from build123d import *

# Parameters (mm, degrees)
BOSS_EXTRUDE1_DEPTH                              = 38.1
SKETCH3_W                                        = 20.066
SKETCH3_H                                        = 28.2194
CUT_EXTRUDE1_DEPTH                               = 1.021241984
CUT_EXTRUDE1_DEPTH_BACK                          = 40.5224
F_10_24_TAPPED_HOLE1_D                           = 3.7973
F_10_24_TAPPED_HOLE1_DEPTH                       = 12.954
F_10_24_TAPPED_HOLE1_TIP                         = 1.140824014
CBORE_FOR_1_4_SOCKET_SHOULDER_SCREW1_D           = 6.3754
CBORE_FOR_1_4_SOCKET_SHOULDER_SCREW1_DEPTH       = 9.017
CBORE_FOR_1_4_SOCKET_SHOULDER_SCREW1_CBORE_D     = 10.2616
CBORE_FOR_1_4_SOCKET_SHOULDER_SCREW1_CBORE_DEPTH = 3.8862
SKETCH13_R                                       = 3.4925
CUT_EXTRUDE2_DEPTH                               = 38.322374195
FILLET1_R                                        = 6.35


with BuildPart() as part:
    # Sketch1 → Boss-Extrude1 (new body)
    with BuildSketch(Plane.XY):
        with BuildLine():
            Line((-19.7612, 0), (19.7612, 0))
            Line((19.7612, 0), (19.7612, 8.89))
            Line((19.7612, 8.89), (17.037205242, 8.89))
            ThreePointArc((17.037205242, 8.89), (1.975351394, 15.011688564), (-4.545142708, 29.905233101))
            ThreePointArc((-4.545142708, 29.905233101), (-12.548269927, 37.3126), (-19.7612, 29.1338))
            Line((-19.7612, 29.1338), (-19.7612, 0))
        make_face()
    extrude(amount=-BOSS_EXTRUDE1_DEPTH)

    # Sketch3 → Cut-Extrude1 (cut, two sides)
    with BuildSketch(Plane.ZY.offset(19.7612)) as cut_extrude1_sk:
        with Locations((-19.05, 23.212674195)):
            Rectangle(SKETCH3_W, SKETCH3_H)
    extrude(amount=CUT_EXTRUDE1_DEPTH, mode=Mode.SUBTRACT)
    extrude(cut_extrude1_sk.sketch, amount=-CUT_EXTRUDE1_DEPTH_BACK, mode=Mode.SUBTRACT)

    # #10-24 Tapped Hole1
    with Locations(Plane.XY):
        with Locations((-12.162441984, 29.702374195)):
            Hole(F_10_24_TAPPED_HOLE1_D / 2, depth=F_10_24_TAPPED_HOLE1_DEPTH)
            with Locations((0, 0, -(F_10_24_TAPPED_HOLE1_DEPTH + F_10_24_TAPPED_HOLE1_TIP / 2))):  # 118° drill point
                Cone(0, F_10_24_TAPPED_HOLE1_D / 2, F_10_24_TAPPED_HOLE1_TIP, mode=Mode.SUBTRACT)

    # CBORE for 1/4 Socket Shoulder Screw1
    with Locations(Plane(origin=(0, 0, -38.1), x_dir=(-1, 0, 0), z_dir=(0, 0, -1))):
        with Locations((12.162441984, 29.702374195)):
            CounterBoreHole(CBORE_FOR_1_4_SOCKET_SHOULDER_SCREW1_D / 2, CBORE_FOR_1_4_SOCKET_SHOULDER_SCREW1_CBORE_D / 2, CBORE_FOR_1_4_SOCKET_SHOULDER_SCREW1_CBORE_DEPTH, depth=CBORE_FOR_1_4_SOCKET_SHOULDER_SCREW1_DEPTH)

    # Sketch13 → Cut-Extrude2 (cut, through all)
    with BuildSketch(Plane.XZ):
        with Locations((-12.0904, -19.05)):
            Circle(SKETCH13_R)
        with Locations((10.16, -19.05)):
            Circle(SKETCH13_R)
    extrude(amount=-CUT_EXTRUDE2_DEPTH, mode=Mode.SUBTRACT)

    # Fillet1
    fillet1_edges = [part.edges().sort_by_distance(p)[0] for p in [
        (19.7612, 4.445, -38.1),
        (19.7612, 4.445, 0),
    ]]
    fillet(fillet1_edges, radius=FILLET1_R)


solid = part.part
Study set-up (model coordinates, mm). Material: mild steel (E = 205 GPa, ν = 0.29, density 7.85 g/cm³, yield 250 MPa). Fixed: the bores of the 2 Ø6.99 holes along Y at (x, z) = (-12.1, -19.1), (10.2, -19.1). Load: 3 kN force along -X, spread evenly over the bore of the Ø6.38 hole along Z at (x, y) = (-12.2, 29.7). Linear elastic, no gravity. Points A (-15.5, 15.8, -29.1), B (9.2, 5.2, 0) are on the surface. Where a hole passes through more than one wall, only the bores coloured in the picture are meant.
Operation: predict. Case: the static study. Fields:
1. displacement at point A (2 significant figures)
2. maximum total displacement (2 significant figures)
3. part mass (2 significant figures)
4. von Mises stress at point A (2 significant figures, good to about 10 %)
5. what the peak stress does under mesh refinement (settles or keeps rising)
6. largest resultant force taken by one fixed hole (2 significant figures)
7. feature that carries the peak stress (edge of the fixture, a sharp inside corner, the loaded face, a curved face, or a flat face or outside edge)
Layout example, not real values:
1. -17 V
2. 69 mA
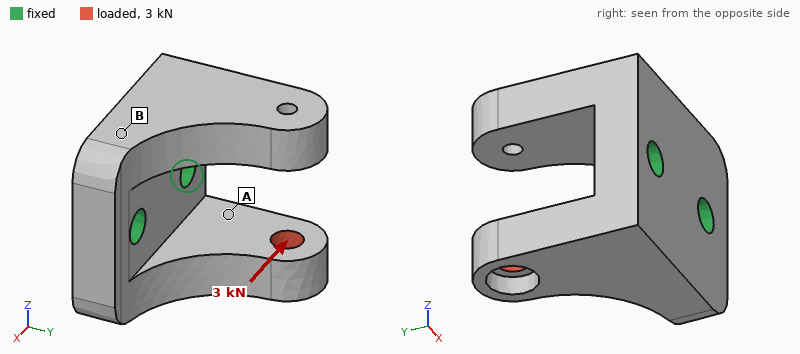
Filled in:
1. 17 µm
2. 51 µm
3. 170 g
4. 61 MPa
5. keeps rising
6. 3.4 kN
7. edge of the fixture
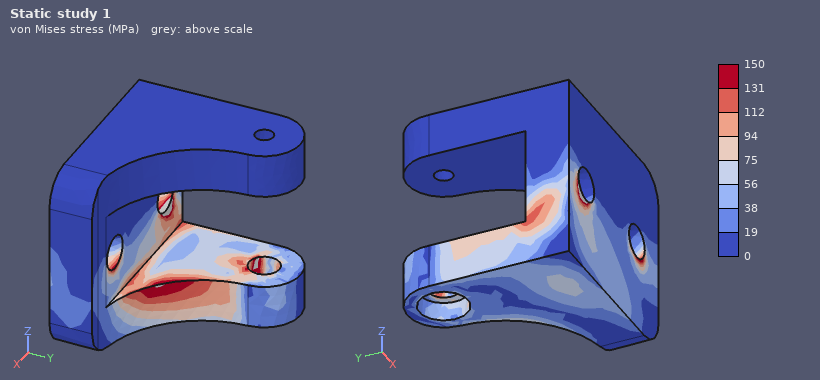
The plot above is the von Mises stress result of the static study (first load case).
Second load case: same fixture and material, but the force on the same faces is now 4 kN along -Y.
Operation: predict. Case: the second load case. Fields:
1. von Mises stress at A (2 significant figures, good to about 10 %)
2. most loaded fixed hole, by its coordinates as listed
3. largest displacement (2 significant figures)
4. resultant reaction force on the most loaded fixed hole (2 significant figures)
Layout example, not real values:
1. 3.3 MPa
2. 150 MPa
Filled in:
1. 66 MPa
2. (-12.1, -19.1)
3. 23 µm
4. 3.6 kN
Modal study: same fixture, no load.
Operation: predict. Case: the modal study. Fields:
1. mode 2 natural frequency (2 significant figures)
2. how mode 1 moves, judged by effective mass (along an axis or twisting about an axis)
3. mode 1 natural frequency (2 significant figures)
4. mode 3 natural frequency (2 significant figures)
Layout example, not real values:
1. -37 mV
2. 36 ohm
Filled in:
1. 6900 Hz
2. along Z
3. 6200 Hz
4. 11 kHz
